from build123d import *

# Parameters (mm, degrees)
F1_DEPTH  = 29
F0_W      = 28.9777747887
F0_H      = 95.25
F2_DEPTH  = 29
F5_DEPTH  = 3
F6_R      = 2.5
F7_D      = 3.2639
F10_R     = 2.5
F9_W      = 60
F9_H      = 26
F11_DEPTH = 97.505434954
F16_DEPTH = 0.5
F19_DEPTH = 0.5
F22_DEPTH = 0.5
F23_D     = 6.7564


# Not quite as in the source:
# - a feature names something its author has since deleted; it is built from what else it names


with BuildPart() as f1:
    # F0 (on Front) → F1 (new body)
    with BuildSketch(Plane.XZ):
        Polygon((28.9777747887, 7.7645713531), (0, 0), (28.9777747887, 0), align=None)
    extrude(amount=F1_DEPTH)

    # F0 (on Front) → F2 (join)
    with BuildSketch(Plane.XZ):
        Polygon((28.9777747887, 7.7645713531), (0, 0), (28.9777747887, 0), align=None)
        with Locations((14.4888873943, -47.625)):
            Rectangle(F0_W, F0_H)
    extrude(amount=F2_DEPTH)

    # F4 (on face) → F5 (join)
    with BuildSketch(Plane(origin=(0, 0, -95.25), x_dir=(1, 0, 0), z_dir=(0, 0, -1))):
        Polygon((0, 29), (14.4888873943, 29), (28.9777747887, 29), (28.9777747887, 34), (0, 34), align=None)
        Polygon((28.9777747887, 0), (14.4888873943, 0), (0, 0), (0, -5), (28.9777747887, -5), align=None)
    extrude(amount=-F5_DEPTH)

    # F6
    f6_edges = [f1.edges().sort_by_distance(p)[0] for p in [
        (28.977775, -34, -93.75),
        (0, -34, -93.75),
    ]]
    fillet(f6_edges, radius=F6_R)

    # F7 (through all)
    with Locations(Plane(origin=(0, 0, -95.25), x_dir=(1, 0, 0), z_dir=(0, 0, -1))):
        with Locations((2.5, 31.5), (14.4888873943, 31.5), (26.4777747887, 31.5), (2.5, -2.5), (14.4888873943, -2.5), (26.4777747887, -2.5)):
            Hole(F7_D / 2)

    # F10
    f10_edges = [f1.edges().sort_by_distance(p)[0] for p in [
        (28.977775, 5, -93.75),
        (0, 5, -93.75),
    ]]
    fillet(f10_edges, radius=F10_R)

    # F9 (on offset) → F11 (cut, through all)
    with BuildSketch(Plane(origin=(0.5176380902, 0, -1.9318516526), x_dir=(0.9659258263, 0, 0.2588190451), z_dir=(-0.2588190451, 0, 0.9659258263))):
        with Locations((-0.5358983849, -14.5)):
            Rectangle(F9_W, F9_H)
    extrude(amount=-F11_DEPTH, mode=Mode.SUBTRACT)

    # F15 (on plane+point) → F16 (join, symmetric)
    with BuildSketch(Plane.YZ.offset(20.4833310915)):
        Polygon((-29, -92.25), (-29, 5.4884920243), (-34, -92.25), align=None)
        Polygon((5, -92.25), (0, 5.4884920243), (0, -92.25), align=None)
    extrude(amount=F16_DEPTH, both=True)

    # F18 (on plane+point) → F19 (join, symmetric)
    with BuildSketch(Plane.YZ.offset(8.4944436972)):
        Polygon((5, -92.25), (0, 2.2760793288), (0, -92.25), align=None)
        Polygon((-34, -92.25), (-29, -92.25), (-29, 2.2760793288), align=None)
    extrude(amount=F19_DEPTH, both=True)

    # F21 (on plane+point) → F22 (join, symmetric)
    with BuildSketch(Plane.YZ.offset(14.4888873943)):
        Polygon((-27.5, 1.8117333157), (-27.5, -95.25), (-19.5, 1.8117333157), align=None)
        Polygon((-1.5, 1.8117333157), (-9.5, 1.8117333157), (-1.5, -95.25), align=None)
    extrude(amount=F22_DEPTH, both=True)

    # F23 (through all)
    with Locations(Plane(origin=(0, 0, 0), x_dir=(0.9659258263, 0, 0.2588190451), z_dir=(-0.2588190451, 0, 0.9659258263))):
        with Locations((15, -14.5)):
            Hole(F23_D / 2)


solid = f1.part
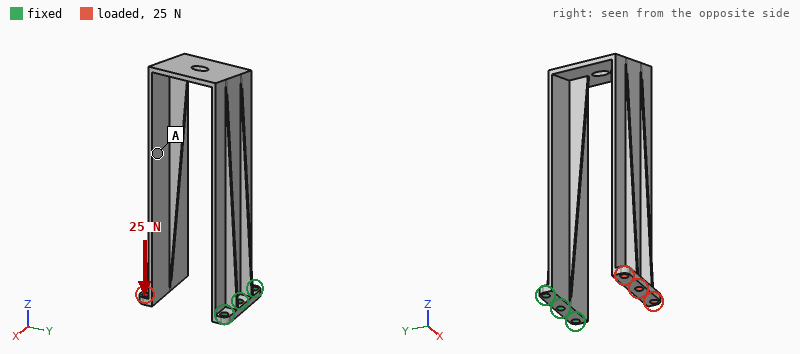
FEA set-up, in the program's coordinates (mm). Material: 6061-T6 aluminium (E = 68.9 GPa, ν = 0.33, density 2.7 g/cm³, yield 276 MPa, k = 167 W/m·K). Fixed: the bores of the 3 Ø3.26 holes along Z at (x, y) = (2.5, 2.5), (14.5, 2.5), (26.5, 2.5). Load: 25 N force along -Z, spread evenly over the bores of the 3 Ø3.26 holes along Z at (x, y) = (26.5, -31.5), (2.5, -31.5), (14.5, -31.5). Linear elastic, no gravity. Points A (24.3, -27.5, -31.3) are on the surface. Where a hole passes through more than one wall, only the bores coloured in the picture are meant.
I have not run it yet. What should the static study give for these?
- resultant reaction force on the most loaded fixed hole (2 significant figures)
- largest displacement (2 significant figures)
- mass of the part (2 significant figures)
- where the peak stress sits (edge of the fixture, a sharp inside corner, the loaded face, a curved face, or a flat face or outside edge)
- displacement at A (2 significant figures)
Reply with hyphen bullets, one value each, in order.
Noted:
- 19 N
- 1.4 mm
- 34 g
- a flat face or outside edge
- 0.43 mm
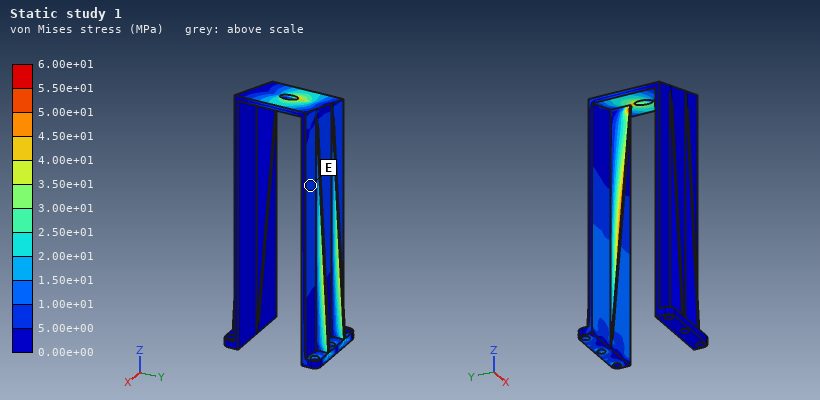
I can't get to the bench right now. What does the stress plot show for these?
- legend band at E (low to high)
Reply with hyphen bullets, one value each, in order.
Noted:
- 5.00e+00 to 1.00e+01 MPa
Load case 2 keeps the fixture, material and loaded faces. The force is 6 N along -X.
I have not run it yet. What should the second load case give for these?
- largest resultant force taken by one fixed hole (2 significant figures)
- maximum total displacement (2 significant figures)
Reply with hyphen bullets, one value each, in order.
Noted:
- 9.3 N
- 1.3 mm
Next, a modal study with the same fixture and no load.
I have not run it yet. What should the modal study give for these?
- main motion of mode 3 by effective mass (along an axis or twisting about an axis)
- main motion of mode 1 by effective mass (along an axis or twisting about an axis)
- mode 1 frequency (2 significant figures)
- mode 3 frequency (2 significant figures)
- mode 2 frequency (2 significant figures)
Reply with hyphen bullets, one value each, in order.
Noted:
- along Y
- along X
- 120 Hz
- 180 Hz
- 140 Hz
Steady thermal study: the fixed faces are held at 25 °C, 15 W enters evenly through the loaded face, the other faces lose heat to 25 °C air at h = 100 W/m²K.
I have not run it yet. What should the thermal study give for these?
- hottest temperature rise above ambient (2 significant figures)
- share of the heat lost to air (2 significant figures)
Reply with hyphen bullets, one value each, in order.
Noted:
- 56 K
- 100 %
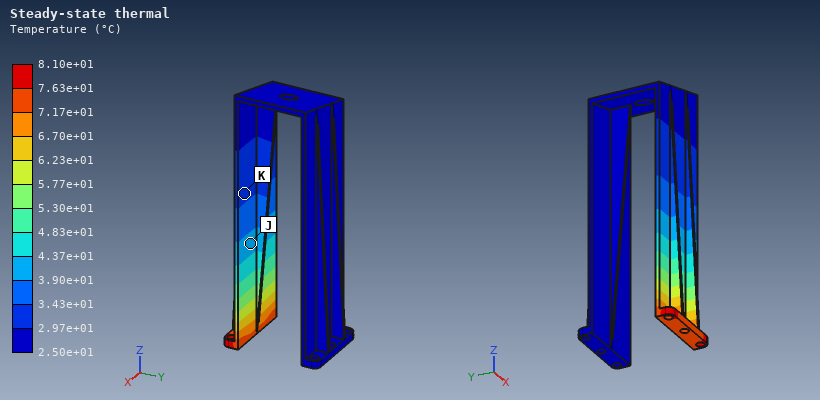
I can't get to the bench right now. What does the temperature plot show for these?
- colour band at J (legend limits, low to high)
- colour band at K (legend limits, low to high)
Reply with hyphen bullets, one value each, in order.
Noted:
- 3.90e+01 to 4.37e+01 °C
- 2.97e+01 to 3.43e+01 °C
